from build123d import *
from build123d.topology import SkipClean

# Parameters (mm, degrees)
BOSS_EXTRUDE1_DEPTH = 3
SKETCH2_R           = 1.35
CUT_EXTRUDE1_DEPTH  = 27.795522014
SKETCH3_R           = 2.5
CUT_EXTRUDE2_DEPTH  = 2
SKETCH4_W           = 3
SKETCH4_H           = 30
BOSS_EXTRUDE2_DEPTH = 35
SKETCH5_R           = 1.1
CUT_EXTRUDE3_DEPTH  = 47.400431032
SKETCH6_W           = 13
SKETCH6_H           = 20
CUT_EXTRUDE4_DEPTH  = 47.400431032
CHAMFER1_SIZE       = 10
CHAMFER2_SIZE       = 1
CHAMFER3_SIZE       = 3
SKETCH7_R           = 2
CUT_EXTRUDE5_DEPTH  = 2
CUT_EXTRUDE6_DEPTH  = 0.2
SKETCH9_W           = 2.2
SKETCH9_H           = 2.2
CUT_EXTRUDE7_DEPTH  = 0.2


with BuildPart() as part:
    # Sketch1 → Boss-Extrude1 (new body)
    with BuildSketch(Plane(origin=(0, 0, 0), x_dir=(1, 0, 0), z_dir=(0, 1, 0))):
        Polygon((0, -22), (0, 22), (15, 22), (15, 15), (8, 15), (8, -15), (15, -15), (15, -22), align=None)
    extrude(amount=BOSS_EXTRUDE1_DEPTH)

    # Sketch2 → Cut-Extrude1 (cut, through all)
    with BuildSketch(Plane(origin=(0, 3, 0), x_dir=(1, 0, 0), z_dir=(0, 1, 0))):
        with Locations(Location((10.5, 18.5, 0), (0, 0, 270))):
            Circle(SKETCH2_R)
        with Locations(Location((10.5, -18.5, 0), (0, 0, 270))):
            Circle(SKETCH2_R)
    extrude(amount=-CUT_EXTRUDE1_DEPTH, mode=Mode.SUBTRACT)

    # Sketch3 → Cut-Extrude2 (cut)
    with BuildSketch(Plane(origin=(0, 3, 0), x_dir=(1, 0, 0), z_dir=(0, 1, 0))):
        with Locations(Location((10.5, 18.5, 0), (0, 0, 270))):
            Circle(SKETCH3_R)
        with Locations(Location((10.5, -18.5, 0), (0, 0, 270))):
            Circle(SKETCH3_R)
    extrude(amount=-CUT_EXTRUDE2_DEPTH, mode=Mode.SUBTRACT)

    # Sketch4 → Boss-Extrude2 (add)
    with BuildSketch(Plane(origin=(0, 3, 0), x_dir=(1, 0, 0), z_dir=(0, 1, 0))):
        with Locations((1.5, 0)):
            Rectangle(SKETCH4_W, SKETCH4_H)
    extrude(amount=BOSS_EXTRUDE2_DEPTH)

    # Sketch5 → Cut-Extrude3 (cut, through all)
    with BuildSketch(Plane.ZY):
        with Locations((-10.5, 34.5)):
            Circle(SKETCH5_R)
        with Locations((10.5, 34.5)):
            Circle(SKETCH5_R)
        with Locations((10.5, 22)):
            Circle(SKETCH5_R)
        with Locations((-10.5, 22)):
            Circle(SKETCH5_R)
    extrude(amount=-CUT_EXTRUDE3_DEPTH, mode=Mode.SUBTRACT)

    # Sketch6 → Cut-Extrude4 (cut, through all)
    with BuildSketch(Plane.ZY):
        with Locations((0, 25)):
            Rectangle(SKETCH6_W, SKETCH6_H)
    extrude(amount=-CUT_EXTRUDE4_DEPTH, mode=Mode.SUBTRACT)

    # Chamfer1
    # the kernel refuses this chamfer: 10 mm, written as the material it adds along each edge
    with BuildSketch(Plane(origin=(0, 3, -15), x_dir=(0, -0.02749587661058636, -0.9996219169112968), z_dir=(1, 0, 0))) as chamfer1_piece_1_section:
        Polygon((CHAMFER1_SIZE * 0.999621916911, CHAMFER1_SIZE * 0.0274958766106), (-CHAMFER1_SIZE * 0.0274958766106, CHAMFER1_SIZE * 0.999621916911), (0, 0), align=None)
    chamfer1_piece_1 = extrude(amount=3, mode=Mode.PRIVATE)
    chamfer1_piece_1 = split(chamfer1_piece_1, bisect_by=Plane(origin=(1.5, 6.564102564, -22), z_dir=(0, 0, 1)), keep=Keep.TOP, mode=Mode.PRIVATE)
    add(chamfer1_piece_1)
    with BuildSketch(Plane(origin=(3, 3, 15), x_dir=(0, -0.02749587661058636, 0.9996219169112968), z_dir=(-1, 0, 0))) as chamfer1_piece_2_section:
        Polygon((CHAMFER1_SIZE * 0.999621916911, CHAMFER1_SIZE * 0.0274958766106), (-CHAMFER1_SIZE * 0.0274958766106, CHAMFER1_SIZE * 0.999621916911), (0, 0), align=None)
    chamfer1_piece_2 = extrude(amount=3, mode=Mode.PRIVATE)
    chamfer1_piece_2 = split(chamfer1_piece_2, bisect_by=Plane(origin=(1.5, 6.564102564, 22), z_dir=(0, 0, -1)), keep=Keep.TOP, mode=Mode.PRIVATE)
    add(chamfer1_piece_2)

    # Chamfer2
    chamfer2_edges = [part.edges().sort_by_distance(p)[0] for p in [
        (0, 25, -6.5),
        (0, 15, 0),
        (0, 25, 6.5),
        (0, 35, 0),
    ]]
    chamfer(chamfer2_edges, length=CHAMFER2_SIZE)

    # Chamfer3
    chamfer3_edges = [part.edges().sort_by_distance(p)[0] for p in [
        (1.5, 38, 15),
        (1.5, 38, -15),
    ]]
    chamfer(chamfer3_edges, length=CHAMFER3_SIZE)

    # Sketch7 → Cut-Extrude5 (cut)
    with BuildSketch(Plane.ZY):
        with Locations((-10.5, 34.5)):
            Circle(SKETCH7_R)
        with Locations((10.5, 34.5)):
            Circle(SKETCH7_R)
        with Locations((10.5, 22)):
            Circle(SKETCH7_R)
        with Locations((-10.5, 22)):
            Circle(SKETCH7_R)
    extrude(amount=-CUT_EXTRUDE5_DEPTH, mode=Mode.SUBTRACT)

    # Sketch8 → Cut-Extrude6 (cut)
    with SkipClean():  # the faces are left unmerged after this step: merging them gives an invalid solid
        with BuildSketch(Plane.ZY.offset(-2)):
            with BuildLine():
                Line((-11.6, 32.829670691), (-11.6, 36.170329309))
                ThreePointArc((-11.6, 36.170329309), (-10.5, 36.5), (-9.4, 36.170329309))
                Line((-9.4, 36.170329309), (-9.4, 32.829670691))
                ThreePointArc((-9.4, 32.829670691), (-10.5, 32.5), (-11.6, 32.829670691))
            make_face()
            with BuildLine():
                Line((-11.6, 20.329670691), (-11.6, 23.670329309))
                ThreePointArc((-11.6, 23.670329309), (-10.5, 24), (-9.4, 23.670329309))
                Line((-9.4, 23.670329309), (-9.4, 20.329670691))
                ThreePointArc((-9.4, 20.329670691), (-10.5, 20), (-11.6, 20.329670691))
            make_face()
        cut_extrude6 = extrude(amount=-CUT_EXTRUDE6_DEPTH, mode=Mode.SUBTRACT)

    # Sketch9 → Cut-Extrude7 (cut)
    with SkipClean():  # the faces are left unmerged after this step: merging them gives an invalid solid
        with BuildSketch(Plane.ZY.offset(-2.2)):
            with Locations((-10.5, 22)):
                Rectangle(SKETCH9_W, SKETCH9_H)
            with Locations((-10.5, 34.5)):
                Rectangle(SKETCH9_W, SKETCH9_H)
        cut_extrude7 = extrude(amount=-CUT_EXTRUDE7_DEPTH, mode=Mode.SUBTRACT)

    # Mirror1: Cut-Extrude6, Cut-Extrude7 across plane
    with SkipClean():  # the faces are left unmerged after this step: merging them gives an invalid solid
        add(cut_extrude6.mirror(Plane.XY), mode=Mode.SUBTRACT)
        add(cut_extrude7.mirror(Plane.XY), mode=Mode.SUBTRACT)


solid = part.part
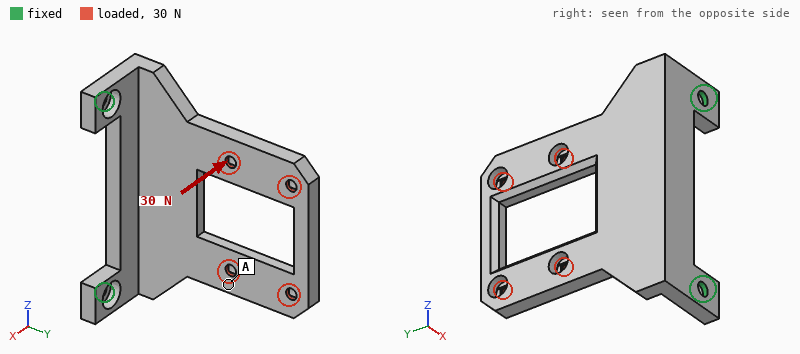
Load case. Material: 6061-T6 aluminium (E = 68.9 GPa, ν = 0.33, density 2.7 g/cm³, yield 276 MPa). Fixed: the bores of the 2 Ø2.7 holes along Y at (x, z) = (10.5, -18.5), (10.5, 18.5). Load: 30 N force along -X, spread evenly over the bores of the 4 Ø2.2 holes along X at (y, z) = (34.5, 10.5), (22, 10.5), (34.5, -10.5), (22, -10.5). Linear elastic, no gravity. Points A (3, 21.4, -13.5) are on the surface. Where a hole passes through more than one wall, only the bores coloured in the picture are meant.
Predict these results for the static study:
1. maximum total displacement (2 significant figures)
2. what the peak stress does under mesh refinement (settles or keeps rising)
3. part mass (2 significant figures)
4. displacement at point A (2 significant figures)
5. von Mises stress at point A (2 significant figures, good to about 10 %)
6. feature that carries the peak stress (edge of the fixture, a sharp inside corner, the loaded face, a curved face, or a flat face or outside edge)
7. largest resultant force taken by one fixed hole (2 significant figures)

0.28 mm
keeps rising
10 g
0.14 mm
11 MPa
edge of the fixture
22 N
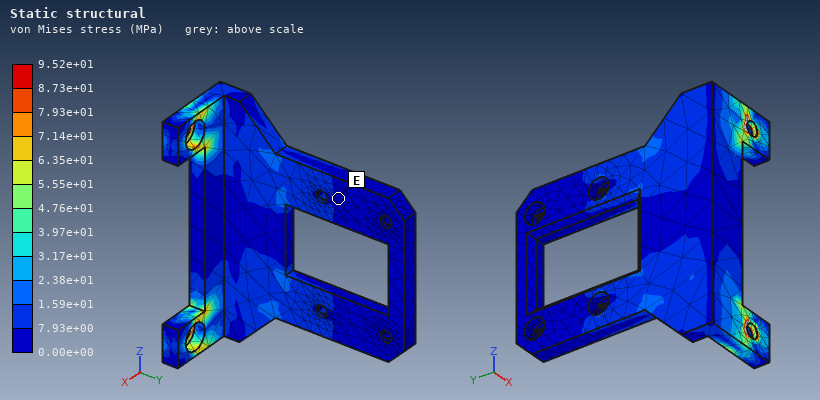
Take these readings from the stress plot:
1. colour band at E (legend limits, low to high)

0.00e+00 to 7.93e+00 MPa
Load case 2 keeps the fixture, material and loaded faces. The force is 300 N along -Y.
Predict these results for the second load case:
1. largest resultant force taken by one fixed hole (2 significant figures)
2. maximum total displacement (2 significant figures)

150 N
0.34 mm
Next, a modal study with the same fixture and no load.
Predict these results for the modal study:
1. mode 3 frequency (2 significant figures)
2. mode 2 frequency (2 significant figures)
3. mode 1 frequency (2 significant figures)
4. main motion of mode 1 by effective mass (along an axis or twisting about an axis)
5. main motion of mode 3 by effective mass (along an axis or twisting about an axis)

4600 Hz
3700 Hz
1100 Hz
along X
along Y
